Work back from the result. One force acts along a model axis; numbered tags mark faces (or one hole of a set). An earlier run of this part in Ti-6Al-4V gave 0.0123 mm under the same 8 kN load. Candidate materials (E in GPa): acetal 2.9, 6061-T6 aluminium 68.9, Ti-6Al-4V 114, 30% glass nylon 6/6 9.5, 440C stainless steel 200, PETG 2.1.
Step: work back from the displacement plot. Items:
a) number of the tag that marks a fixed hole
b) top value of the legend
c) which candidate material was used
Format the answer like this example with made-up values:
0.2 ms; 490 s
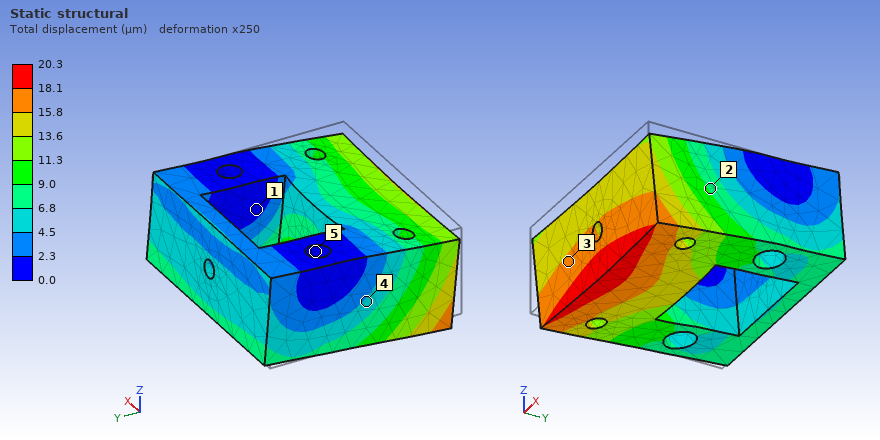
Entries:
5; 20.3 µm; 6061-T6 aluminium
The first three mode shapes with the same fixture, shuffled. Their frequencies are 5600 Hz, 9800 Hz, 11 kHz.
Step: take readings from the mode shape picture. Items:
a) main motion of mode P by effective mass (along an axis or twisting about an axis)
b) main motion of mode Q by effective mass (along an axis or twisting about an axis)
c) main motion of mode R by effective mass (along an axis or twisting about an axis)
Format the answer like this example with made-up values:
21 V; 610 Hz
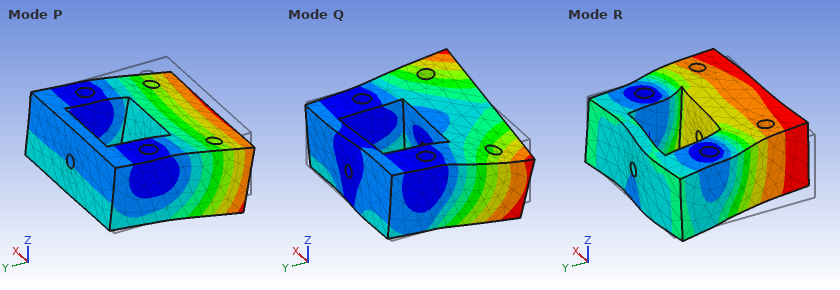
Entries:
along Z; twisting about Y; along X
